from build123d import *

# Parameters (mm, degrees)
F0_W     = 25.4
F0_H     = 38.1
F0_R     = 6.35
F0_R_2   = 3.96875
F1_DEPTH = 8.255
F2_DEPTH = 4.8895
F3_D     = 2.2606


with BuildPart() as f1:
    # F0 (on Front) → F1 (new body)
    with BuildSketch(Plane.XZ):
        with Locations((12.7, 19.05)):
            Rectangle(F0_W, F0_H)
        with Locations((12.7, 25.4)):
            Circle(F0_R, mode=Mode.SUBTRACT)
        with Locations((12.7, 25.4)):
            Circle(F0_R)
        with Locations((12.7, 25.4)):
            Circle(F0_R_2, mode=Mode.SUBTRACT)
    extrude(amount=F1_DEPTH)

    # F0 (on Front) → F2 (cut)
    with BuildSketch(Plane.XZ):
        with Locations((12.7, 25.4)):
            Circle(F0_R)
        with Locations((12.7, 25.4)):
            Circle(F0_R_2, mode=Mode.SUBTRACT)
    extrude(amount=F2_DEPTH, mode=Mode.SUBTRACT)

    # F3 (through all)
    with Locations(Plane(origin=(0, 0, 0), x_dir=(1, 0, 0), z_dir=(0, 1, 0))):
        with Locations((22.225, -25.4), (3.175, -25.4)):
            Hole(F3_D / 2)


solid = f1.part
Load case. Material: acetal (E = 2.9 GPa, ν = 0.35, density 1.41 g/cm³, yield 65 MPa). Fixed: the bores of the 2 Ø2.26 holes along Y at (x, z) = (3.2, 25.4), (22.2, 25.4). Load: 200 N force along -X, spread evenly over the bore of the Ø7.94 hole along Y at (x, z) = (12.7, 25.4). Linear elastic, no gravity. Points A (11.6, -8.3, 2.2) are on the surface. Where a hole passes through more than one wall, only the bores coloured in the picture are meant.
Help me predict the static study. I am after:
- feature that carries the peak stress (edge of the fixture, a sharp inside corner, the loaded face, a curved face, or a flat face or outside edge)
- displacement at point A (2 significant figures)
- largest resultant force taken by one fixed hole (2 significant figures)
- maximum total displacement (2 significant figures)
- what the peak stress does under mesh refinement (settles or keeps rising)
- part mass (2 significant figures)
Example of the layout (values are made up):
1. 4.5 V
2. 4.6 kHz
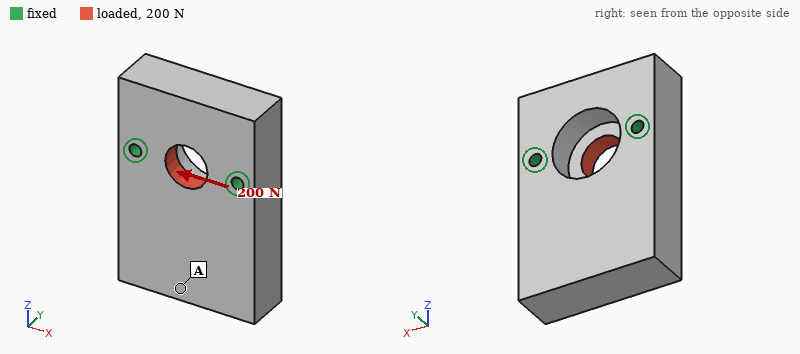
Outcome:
1. edge of the fixture
2. 4.0 µm
3. 100 N
4. 8.7 µm
5. keeps rising
6. 10 g
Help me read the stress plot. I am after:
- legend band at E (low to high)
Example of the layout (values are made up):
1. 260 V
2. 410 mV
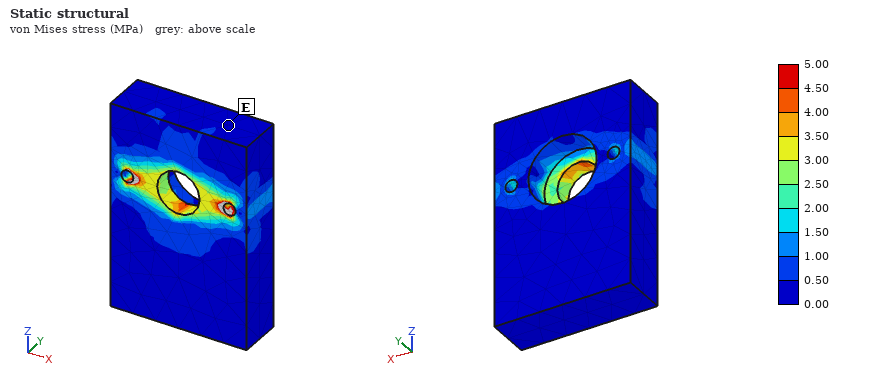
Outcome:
1. 0.00 to 0.50 MPa
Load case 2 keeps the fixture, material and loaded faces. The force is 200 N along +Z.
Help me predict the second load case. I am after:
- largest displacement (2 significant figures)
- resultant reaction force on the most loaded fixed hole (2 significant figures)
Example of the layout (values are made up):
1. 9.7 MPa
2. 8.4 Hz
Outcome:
1. 22 µm
2. 100 N
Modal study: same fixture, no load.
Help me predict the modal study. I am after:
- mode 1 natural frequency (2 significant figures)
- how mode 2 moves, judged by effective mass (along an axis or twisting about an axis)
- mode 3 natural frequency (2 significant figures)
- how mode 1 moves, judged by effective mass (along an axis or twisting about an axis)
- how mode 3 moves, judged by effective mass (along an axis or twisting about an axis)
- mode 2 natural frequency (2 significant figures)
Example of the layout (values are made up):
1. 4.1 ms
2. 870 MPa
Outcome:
1. 2200 Hz
2. along X
3. 5400 Hz
4. along Y
5. along X
6. 5200 Hz
